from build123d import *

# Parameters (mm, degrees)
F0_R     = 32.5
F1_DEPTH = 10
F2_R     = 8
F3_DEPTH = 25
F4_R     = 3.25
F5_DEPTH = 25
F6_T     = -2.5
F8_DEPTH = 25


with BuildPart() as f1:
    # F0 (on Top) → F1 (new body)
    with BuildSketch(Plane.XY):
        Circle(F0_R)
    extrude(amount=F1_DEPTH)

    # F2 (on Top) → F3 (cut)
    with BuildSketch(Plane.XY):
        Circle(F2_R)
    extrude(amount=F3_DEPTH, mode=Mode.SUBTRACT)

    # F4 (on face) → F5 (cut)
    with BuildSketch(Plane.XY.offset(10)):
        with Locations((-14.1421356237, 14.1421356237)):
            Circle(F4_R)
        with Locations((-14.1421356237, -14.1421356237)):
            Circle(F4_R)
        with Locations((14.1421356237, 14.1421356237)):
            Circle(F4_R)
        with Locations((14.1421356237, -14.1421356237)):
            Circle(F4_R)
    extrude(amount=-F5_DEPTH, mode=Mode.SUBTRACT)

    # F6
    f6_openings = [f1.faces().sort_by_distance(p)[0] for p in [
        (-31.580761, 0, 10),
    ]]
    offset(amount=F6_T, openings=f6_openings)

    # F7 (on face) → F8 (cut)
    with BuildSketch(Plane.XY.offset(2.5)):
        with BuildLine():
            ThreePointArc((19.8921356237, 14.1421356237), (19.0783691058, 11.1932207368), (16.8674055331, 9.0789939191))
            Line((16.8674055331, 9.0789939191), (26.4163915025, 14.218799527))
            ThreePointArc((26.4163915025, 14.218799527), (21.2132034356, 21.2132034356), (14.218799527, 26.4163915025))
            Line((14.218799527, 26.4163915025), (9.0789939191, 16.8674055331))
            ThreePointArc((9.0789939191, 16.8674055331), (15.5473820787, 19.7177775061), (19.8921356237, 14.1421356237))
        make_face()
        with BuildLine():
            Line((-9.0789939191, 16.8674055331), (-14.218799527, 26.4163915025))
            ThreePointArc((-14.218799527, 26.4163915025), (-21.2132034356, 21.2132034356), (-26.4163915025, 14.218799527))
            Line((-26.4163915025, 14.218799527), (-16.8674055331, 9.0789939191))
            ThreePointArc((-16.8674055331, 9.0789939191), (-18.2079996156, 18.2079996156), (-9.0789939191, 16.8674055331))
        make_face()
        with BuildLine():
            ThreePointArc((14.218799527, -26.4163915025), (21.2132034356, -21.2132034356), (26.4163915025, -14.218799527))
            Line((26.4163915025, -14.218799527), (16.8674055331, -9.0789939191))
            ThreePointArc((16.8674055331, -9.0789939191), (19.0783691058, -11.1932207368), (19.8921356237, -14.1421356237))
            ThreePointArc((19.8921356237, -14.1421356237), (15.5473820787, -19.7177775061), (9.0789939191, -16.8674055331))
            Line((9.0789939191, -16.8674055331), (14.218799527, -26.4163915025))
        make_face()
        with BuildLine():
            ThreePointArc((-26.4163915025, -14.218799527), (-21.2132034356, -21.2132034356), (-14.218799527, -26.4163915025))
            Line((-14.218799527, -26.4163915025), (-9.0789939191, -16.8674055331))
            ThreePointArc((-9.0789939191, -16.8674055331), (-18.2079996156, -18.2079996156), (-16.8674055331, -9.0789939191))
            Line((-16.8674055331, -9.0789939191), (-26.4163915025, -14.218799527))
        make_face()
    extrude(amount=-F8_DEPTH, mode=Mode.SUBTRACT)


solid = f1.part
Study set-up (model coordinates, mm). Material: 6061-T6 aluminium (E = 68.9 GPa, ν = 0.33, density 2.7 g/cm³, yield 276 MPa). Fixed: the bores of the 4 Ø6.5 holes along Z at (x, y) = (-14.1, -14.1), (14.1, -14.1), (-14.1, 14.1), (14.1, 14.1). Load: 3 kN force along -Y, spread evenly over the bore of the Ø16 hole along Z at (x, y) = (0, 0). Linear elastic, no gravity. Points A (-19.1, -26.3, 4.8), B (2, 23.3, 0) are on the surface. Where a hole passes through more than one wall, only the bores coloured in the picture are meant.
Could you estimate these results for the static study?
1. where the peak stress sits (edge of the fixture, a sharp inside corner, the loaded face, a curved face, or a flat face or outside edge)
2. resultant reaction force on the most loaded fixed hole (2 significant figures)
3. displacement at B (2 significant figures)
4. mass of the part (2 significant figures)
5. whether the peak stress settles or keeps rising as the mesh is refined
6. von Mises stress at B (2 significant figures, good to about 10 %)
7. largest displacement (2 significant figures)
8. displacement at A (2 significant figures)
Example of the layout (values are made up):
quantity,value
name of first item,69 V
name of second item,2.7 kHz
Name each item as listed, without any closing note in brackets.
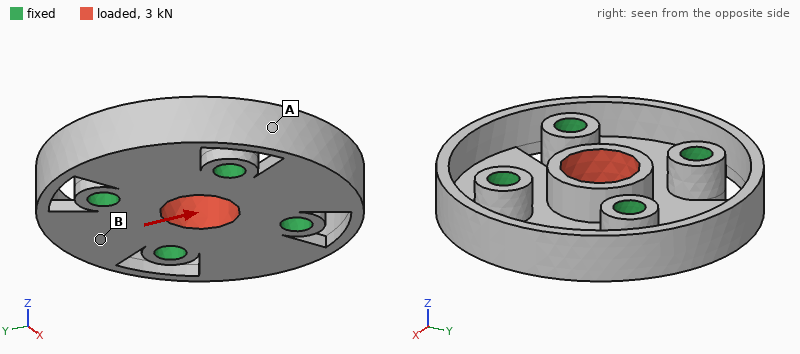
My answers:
quantity,value
where the peak stress sits,edge of the fixture
resultant reaction force on the most loaded fixed hole,810 N
displacement at B,3.8 µm
mass of the part,36 g
whether the peak stress settles or keeps rising as the mesh is refined,keeps rising
von Mises stress at B,10 MPa
largest displacement,22 µm
displacement at A,3.6 µm
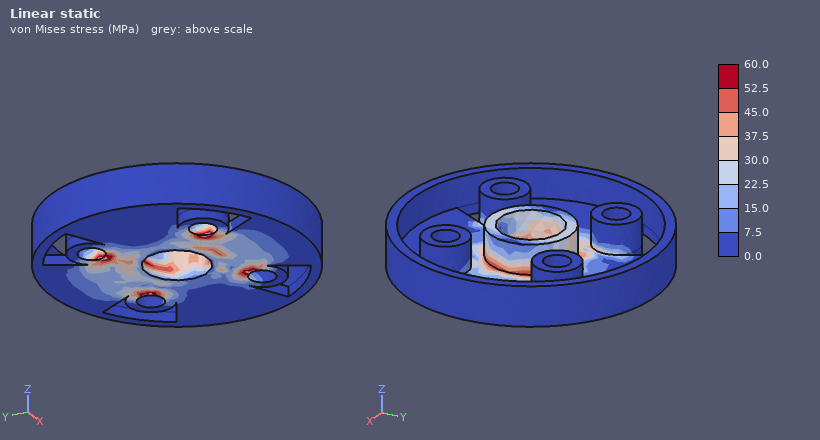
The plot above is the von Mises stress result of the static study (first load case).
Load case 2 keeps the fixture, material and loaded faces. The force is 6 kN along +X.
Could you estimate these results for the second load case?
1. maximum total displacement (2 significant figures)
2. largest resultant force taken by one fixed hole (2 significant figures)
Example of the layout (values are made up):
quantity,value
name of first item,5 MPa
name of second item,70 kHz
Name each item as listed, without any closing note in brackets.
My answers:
quantity,value
maximum total displacement,44 µm
largest resultant force taken by one fixed hole,1.6 kN
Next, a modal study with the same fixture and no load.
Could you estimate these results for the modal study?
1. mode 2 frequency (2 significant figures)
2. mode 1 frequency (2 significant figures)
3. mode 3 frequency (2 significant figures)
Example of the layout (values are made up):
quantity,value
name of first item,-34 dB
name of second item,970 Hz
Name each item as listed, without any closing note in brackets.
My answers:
quantity,value
mode 2 frequency,3900 Hz
mode 1 frequency,3900 Hz
mode 3 frequency,4400 Hz
